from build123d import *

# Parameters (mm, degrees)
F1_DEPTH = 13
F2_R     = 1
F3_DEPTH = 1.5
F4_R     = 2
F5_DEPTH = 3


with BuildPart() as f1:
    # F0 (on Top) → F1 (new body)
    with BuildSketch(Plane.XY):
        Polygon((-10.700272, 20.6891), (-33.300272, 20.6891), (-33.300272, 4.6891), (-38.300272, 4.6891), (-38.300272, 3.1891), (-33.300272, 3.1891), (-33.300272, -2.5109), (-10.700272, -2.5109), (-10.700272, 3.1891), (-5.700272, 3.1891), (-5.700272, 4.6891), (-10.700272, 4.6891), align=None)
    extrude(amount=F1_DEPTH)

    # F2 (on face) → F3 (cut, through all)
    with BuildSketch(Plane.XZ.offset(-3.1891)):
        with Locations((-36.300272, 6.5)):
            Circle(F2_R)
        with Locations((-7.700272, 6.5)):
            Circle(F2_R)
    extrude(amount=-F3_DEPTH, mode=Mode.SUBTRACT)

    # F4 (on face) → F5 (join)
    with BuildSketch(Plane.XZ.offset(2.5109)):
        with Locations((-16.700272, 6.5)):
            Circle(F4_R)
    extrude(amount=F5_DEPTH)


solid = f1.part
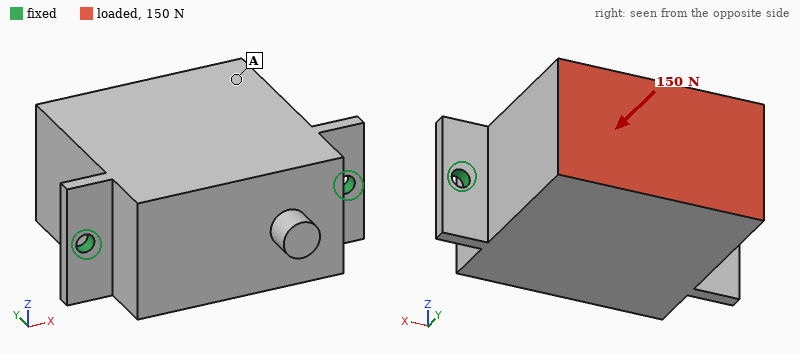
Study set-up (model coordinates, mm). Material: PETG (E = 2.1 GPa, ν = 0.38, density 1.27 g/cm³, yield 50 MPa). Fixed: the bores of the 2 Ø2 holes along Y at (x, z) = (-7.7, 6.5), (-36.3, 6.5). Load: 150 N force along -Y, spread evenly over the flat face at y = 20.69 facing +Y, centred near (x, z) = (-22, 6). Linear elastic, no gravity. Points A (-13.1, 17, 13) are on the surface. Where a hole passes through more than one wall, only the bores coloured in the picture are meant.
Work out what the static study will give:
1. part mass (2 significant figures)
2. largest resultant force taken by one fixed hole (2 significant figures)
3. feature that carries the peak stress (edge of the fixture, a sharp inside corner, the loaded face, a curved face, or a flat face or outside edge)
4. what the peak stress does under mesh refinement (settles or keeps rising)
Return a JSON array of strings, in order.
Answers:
["8.9 g", "75 N", "edge of the fixture", "keeps rising"]
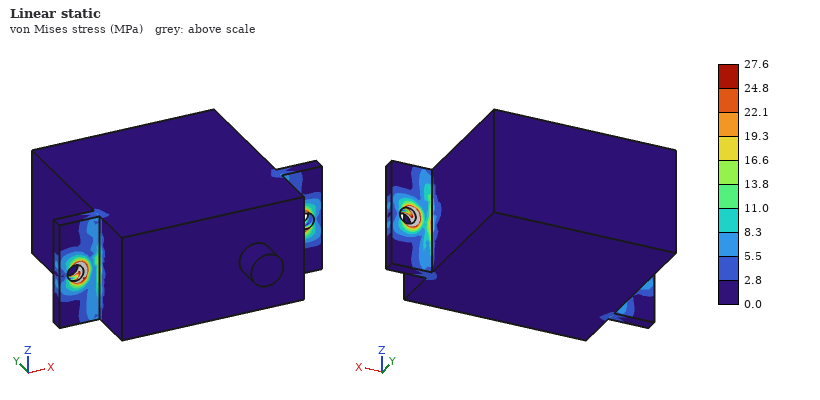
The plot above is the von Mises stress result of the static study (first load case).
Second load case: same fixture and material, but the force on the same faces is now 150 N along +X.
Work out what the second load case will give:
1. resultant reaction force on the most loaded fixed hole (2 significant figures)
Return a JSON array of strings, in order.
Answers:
["120 N"]
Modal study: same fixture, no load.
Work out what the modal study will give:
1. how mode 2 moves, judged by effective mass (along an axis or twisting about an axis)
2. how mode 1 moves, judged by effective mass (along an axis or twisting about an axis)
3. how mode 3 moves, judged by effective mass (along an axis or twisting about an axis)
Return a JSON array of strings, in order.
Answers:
["along Y", "along Z", "along X"]
